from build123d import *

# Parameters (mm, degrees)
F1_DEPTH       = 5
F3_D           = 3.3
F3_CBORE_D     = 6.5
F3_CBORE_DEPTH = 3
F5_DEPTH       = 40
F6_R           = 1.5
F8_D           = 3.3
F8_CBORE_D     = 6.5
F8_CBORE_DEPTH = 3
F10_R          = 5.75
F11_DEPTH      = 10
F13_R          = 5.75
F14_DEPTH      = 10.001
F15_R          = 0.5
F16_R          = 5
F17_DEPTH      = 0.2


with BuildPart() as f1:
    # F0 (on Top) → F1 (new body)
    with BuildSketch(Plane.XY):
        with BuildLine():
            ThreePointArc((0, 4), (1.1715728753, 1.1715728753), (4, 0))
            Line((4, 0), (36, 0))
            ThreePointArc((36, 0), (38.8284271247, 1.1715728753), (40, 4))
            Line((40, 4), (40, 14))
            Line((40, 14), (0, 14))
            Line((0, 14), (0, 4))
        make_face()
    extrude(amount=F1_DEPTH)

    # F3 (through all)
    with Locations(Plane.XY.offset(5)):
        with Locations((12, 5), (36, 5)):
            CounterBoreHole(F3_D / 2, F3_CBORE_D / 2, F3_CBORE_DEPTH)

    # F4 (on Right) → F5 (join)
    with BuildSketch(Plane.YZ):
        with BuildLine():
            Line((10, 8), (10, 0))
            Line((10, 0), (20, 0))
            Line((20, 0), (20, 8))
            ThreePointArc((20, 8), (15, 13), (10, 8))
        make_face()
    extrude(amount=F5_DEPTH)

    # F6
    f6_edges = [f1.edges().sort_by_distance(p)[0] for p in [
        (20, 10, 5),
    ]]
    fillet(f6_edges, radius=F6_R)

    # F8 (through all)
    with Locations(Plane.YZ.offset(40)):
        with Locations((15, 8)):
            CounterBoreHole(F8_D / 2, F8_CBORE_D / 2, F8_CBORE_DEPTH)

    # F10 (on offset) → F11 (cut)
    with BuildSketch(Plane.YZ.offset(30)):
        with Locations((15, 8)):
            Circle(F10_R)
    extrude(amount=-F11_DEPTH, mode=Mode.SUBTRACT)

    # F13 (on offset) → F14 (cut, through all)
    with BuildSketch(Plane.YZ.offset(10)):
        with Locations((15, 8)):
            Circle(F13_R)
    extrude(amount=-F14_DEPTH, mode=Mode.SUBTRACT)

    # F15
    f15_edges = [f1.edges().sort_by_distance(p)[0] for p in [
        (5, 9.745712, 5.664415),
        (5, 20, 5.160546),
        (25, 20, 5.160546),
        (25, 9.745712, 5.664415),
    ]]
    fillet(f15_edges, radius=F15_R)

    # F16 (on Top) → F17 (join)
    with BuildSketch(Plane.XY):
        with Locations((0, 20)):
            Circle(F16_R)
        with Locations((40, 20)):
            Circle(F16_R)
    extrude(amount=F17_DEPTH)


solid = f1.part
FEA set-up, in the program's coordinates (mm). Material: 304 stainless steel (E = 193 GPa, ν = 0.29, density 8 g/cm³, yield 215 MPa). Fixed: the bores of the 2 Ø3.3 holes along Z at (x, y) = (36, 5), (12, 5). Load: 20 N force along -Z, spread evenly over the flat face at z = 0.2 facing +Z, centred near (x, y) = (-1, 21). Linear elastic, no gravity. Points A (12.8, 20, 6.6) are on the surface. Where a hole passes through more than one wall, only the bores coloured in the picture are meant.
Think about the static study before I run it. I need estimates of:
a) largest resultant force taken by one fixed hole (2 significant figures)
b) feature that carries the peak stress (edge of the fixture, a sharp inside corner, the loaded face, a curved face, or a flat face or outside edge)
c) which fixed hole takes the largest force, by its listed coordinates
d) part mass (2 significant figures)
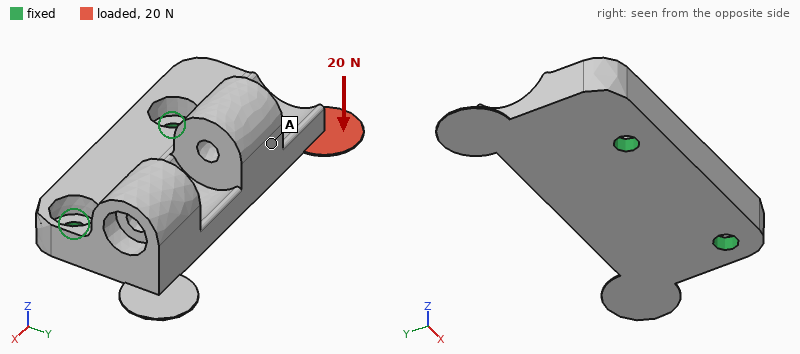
31 N
a flat face or outside edge
(12, 5)
36 g
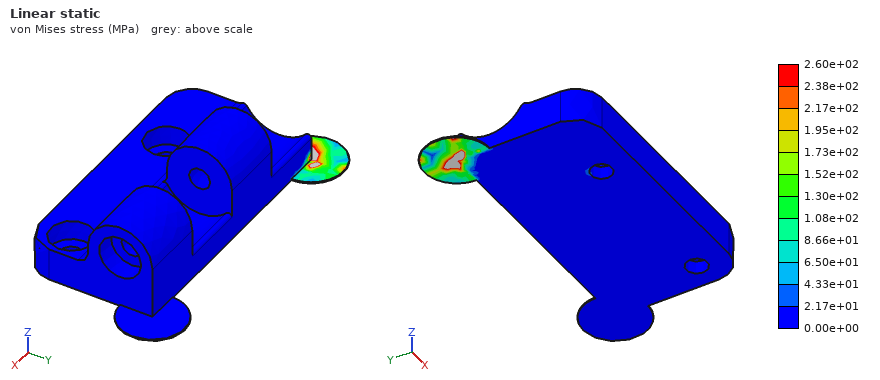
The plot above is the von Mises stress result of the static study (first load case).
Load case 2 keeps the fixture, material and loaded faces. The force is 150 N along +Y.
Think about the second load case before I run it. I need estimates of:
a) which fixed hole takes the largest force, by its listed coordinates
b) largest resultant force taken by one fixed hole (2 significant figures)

(12, 5)
220 N
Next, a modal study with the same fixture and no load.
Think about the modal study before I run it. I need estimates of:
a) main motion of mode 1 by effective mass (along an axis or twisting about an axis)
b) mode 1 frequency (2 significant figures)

along Z
5300 Hz
